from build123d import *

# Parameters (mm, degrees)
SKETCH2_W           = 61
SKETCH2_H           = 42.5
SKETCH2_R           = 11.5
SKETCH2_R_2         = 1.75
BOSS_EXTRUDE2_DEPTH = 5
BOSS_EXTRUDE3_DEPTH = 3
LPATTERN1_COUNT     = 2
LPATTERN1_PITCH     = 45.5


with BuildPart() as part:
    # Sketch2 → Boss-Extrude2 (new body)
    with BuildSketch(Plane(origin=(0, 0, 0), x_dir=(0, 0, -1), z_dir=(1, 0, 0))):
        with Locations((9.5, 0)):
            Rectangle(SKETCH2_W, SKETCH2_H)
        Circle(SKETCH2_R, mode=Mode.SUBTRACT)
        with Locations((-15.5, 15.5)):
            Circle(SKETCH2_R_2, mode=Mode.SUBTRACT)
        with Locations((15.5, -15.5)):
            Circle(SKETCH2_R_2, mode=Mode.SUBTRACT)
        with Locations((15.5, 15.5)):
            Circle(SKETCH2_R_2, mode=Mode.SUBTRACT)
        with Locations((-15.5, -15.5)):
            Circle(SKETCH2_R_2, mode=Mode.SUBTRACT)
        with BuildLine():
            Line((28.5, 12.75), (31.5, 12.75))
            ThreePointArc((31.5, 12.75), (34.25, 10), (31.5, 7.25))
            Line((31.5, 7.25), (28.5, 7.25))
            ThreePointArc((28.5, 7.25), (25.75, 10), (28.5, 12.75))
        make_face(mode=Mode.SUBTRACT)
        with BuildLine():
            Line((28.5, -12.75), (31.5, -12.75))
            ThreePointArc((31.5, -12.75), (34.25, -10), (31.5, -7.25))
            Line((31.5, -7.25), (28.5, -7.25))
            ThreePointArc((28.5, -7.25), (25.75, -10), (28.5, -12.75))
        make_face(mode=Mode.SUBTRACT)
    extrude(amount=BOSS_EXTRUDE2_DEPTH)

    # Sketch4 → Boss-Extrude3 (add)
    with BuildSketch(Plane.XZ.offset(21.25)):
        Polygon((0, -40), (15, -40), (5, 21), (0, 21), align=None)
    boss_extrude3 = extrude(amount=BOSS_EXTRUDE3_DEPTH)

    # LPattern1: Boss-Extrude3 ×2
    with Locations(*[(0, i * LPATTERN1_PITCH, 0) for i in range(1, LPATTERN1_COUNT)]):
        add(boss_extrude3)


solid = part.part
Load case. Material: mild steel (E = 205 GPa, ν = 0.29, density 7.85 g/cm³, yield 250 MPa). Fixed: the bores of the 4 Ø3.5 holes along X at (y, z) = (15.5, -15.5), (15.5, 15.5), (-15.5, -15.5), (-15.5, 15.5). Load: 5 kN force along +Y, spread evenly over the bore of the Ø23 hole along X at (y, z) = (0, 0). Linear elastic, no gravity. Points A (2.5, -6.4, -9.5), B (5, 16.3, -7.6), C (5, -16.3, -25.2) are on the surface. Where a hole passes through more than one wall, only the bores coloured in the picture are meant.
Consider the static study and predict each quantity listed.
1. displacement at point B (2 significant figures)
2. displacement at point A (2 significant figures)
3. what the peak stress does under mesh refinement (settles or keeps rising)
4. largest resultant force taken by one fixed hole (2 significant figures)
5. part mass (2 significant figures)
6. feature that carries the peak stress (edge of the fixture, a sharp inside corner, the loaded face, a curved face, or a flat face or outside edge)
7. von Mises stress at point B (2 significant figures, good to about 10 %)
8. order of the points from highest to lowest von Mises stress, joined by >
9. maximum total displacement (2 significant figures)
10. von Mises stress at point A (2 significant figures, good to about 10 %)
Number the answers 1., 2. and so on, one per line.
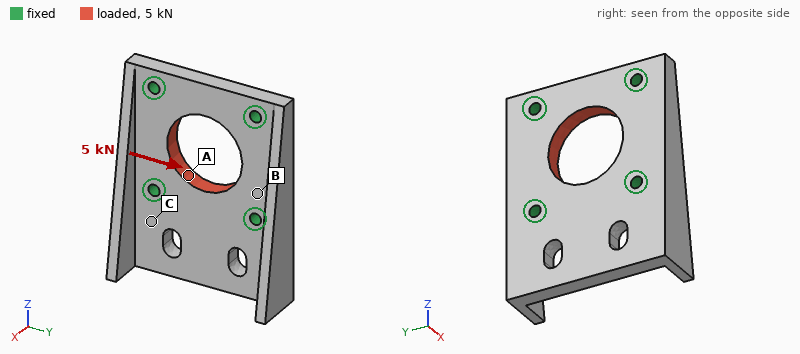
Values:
1. 1.4 µm
2. 1.3 µm
3. keeps rising
4. 1.3 kN
5. 110 g
6. edge of the fixture
7. 16 MPa
8. A > B > C
9. 2.4 µm
10. 28 MPa
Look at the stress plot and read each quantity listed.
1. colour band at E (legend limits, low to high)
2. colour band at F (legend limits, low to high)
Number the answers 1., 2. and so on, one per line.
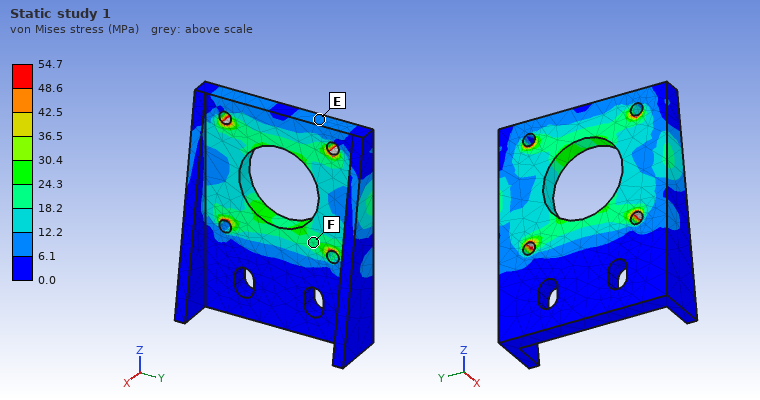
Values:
1. 6.1 to 12.2 MPa
2. 18.2 to 24.3 MPa
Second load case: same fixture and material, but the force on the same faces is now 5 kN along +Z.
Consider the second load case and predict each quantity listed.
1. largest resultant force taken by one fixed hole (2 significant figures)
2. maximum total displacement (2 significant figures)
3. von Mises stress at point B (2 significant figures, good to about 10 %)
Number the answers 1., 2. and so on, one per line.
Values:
1. 1.3 kN
2. 3.1 µm
3. 14 MPa
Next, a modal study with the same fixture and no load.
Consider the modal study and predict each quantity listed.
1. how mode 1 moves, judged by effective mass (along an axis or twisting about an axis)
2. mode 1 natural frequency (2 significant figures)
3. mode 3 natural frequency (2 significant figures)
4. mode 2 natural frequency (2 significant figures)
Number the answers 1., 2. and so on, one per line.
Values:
1. along X
2. 7000 Hz
3. 11 kHz
4. 8800 Hz
